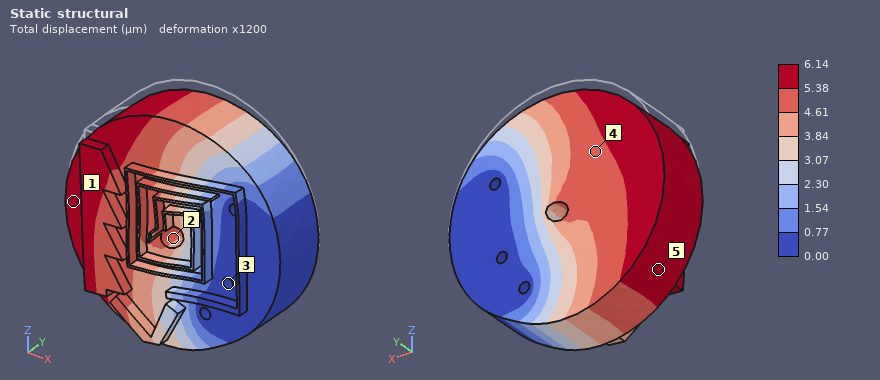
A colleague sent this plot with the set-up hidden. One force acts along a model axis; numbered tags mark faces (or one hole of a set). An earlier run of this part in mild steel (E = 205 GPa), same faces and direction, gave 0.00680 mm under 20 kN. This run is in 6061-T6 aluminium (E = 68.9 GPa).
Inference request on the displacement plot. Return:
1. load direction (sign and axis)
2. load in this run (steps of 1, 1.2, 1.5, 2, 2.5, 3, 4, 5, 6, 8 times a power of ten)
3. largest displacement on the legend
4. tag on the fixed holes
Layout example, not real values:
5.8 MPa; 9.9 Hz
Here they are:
-Z; 6 kN; 6.14 µm; 3
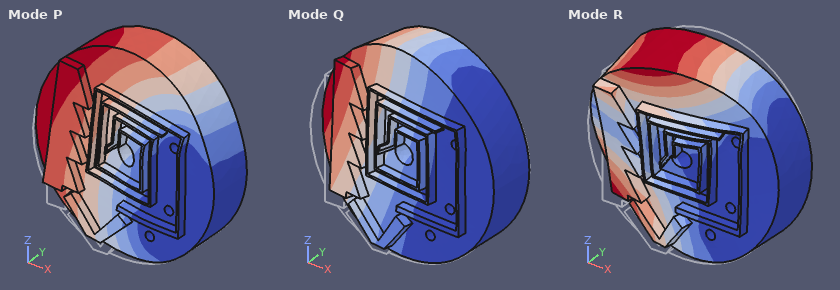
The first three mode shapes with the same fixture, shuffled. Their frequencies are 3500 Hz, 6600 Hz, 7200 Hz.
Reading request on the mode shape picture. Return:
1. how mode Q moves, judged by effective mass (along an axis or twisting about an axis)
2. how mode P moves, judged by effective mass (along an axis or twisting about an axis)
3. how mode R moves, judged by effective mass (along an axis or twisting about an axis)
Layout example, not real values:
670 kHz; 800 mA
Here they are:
along Y; along Z; twisting about X
